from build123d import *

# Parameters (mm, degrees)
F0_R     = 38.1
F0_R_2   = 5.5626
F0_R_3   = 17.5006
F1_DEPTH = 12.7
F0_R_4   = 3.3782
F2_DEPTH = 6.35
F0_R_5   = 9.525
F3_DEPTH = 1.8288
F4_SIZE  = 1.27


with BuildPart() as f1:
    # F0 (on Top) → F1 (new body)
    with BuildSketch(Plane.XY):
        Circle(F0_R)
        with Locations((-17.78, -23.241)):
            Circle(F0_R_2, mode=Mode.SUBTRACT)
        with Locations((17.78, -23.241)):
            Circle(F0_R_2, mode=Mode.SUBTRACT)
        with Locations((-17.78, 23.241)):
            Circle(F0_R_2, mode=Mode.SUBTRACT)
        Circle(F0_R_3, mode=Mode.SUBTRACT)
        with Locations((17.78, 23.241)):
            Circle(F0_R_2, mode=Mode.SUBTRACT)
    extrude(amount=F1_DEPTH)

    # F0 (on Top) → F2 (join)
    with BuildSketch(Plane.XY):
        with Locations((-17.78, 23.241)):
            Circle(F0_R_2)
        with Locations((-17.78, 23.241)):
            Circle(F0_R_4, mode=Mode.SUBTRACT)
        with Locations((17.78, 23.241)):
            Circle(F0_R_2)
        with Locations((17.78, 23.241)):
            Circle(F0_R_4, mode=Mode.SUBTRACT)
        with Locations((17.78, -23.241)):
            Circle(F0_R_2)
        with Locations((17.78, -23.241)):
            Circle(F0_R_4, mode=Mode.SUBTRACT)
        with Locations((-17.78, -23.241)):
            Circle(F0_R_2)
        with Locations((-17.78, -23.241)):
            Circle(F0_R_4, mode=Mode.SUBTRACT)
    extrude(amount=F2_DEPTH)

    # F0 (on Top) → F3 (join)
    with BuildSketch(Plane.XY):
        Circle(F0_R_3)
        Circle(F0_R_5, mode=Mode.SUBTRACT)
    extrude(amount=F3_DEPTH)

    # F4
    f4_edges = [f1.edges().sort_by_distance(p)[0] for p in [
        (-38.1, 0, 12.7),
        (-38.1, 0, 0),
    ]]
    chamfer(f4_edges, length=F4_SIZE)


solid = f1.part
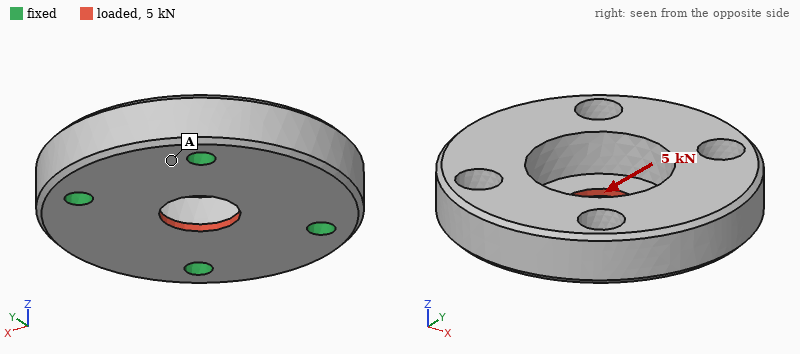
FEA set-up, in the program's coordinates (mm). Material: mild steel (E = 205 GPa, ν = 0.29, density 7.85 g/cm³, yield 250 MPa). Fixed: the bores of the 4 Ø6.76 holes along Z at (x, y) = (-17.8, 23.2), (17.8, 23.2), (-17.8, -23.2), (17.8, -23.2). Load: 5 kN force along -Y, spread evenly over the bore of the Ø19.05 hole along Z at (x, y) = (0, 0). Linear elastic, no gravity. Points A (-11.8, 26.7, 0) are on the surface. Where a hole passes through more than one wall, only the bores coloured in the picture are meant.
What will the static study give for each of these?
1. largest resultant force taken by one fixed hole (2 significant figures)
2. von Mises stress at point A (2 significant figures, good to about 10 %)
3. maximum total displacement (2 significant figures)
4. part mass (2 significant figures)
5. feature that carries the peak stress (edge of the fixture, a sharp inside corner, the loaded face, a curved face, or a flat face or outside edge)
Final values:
1.3 kN
11 MPa
3.9 µm
340 g
the loaded face
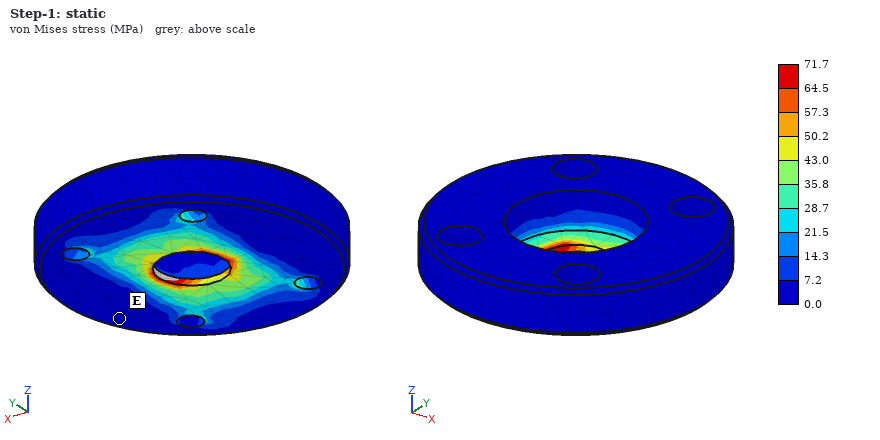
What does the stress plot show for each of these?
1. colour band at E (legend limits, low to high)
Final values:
0.0 to 7.2 MPa
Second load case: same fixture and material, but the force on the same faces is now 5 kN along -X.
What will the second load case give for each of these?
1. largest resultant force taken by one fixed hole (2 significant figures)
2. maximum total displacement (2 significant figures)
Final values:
1.3 kN
4.6 µm
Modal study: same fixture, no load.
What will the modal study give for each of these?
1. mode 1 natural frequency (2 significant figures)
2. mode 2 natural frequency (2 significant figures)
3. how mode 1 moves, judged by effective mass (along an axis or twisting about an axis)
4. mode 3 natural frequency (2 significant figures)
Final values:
12 kHz
13 kHz
along Z
20 kHz
